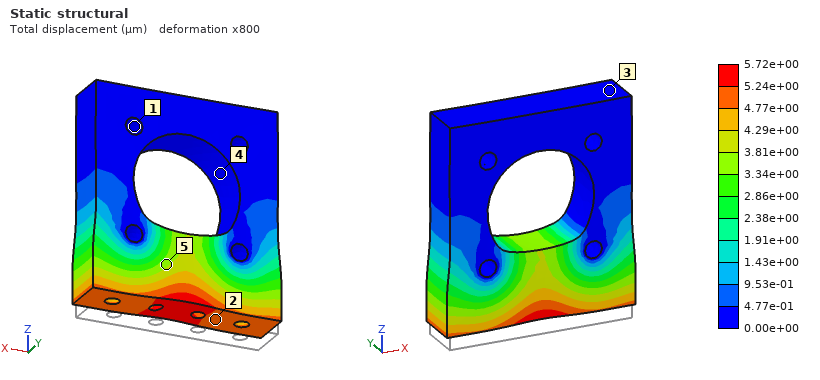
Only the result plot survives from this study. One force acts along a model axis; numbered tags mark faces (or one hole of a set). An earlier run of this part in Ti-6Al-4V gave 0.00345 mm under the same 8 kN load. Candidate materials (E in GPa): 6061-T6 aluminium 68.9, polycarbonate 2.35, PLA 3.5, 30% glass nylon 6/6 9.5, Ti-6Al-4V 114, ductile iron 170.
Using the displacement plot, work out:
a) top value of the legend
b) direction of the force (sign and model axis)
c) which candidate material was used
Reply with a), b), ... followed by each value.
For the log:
a) 5.72e+00 µm
b) +Z
c) 6061-T6 aluminium
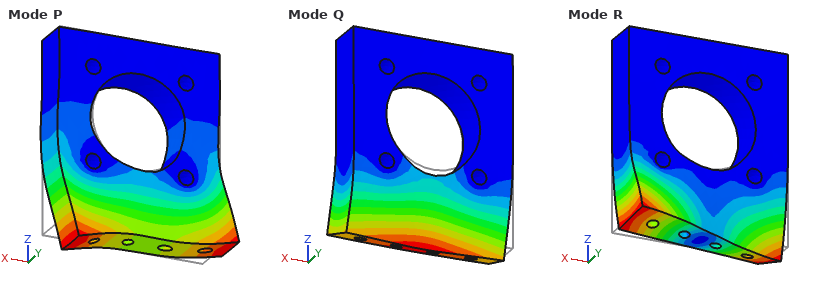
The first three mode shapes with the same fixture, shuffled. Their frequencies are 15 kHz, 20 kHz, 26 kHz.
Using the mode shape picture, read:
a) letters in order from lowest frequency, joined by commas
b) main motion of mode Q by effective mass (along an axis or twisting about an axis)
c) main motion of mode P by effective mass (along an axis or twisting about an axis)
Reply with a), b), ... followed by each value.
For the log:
a) Q, R, P
b) along Y
c) along X
